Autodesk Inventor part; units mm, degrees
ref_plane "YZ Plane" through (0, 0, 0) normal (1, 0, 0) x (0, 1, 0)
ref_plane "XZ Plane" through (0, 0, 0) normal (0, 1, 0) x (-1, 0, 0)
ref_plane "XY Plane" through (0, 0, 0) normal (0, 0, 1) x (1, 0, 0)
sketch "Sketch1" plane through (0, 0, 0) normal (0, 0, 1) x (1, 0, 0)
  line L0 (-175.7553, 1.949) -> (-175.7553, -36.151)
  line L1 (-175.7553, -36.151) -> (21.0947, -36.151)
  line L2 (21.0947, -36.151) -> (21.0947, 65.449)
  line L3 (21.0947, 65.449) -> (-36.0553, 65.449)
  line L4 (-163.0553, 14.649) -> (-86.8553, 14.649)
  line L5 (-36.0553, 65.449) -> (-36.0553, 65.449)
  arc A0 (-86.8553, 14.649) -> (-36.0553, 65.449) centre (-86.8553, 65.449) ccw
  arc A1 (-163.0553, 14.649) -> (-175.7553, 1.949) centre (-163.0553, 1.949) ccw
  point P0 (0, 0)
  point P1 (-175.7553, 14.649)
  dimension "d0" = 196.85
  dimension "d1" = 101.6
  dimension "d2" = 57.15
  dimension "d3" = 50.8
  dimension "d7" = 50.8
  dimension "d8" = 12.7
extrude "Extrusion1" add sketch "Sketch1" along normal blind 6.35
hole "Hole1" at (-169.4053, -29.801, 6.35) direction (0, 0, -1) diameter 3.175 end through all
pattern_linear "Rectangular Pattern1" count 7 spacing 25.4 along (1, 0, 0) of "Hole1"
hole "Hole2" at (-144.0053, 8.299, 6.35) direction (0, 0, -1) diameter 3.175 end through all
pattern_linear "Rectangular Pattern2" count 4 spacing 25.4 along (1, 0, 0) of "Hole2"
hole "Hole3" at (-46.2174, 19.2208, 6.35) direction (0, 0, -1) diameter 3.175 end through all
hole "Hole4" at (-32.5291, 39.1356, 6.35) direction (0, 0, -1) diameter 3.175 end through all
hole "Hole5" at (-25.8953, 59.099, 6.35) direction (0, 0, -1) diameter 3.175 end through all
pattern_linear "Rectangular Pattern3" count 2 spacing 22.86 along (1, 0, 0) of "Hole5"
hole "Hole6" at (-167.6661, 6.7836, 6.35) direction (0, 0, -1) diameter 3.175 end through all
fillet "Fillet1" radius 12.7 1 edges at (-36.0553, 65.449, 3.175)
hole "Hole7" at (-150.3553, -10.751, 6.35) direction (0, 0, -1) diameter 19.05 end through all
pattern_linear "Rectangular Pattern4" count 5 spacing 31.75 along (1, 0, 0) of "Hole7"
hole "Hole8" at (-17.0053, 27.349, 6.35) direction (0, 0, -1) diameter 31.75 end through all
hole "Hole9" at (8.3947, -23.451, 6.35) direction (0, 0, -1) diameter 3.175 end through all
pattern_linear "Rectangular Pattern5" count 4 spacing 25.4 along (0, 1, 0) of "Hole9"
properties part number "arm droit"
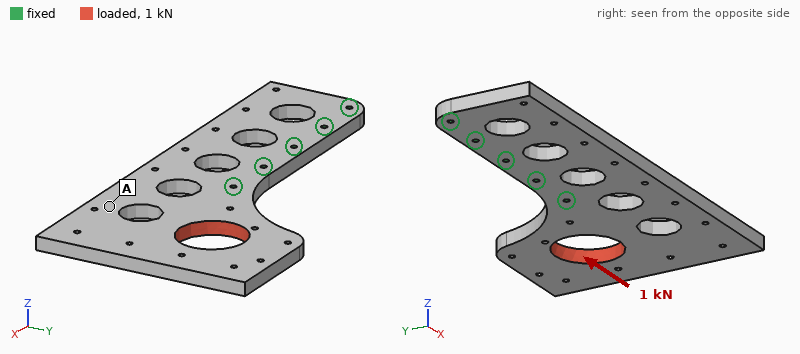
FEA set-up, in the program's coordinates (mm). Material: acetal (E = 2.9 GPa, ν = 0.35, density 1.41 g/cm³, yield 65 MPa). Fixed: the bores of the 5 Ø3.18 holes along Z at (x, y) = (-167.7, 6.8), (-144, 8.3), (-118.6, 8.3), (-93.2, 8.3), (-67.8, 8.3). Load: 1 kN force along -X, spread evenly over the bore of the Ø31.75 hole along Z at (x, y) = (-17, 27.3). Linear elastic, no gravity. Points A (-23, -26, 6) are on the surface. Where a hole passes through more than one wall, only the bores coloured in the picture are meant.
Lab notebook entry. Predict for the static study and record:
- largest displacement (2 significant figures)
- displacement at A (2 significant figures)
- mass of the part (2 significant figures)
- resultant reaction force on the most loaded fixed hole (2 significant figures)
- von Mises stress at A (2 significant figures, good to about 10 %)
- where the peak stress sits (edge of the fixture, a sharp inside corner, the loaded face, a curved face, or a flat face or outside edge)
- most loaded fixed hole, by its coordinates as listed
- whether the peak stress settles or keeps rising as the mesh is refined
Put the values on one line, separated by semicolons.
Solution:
1.0 mm; 0.37 mm; 99 g; 1.2 kN; 2.6 MPa; edge of the fixture; (-67.8, 8.3); keeps rising
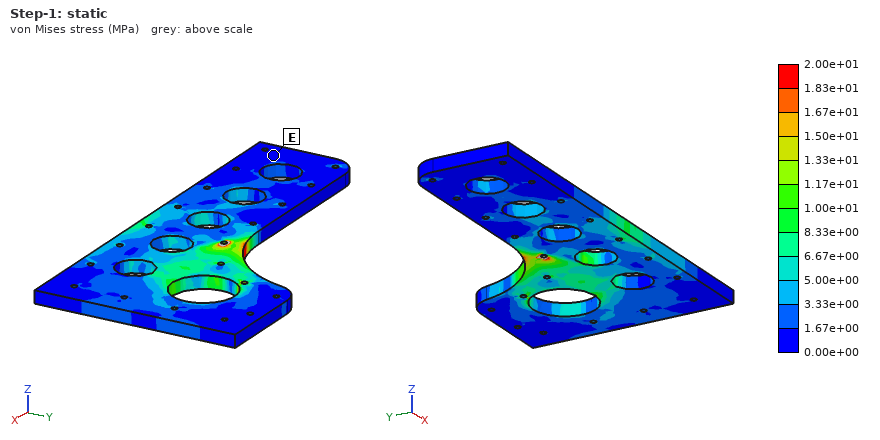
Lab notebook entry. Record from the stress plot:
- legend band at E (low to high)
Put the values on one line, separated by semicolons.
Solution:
0.00e+00 to 1.67e+00 MPa
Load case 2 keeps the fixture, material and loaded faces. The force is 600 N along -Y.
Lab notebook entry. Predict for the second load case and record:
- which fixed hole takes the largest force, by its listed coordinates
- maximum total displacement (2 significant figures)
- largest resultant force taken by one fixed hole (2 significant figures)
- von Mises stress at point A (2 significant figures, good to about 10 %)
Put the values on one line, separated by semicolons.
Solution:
(-67.8, 8.3); 1.2 mm; 1.1 kN; 4.6 MPa
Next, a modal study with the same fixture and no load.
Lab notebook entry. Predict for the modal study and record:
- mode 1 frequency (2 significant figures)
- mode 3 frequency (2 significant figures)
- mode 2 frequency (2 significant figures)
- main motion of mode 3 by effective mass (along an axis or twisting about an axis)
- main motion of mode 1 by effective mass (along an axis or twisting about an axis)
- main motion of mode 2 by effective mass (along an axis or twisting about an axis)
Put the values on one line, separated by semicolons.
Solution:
120 Hz; 550 Hz; 200 Hz; along Y; along Z; twisting about X
